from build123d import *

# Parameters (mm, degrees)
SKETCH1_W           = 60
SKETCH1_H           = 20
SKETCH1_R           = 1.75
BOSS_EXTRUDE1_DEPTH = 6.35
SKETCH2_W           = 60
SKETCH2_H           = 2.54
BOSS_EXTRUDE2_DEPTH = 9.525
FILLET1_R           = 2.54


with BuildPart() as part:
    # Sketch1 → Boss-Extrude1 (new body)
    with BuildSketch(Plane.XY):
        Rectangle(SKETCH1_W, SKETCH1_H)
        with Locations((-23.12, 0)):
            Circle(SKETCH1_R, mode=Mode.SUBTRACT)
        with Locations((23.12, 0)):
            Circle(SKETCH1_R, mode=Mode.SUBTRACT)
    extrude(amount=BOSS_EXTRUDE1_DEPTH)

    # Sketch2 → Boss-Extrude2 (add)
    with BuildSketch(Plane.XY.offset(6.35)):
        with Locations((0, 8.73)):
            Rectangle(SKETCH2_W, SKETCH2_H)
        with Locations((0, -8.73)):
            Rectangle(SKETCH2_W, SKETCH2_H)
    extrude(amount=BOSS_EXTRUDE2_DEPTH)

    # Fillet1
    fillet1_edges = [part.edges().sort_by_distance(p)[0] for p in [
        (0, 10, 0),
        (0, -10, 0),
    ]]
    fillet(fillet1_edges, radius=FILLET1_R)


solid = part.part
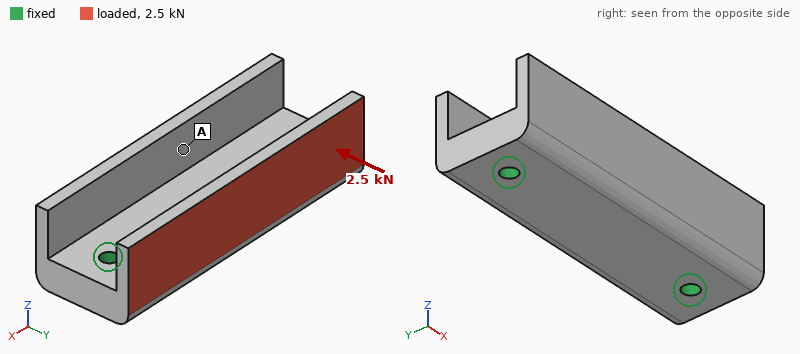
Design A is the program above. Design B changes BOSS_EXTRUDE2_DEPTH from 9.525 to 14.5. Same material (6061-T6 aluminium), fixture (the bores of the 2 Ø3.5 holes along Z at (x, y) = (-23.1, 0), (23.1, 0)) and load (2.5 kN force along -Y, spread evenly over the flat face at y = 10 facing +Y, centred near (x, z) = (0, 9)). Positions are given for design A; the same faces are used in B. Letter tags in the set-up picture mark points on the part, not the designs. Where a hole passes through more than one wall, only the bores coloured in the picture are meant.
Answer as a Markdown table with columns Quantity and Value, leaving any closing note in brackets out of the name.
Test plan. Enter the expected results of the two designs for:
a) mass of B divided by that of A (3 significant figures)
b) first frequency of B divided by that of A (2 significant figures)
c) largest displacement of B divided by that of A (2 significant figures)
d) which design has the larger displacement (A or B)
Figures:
| Quantity | Value |
|---|---|
| mass of B divided by that of A | 1.15 |
| first frequency of B divided by that of A | 0.64 |
| largest displacement of B divided by that of A | 2.5 |
| which design has the larger displacement | B |
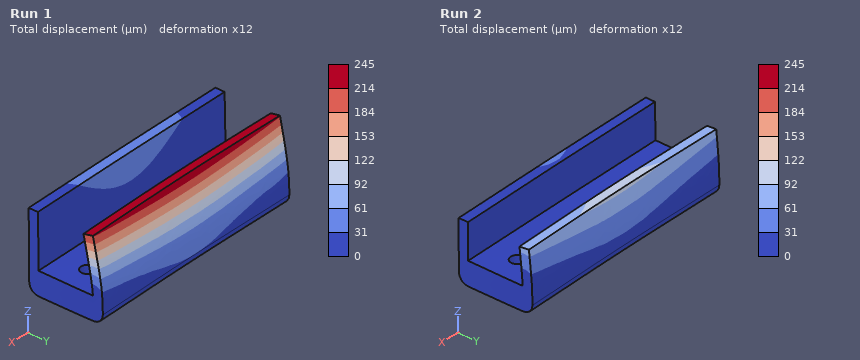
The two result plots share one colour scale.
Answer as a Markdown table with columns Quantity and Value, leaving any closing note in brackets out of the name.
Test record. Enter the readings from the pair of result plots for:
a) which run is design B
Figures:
| Quantity | Value |
|---|---|
| which run is design B | Run 1 |
